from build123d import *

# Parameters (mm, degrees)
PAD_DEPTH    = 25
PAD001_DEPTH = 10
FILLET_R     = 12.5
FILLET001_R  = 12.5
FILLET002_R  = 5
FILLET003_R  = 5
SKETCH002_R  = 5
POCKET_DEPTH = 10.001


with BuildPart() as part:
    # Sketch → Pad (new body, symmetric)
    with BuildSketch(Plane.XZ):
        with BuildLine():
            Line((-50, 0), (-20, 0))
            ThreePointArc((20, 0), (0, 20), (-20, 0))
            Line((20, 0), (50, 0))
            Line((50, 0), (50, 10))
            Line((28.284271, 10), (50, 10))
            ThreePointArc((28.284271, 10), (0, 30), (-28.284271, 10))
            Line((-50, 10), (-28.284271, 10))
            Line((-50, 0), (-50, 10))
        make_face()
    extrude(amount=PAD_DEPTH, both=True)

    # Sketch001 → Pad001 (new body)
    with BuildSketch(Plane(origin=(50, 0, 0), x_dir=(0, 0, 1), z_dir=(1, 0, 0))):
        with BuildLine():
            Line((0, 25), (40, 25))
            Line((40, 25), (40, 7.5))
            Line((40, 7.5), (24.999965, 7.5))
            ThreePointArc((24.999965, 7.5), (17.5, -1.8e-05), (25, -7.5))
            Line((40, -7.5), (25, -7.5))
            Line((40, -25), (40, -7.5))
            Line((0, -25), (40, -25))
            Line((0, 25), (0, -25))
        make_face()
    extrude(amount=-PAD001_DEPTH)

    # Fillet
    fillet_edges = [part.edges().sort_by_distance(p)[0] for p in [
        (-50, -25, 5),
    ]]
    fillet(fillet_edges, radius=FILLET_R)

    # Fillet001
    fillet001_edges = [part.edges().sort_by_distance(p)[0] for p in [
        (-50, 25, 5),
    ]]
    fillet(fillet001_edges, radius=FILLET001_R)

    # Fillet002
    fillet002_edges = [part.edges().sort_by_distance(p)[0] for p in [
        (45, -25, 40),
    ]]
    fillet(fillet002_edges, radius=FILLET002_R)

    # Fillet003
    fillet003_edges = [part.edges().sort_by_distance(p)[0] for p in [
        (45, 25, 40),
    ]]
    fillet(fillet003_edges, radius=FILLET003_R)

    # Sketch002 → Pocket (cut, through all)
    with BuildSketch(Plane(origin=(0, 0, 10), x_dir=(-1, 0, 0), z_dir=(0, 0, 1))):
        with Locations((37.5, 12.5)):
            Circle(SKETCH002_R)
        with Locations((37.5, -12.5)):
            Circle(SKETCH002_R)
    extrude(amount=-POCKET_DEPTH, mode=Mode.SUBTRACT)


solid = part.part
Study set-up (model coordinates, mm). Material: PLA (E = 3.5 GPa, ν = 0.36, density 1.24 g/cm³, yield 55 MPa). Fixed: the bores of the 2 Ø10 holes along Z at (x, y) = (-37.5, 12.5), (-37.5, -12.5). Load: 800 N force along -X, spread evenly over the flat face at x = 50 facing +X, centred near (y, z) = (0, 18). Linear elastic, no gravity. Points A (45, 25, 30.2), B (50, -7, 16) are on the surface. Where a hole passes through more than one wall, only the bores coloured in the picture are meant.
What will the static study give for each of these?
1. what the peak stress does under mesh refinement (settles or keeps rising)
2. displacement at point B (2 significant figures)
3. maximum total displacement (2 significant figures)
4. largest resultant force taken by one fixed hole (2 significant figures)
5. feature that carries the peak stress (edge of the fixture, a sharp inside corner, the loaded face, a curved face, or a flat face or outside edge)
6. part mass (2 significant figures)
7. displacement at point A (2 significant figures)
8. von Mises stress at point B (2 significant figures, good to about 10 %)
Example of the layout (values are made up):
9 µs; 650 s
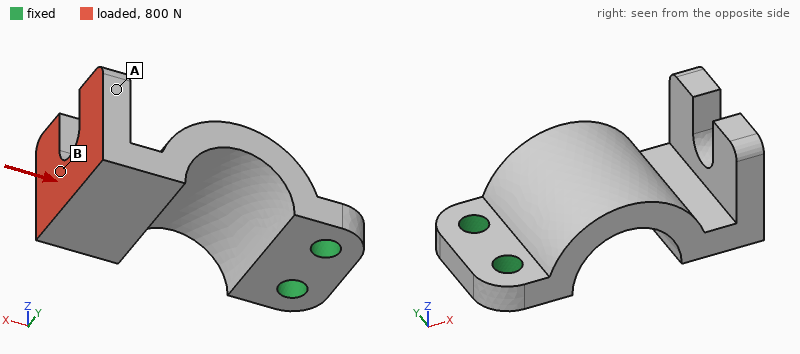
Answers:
keeps rising; 0.78 mm; 1.2 mm; 410 N; edge of the fixture; 86 g; 0.92 mm; 6.9 MPa
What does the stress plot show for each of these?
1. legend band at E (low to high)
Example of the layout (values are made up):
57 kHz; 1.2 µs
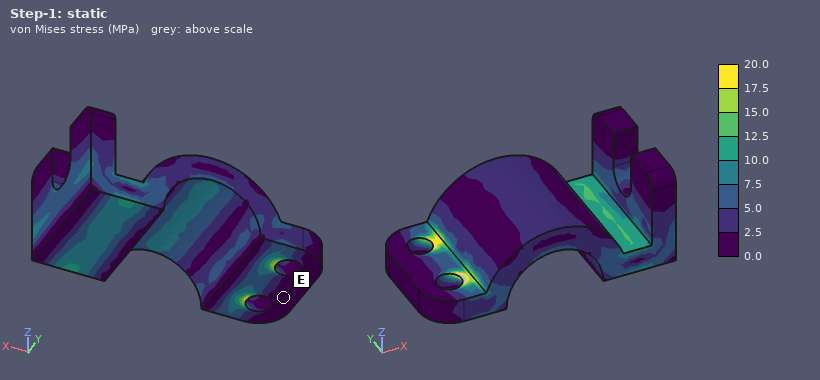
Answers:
0.0 to 2.5 MPa
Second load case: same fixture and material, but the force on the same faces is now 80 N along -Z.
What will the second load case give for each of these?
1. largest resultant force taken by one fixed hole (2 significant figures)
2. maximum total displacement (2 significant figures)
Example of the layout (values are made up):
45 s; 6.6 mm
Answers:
41 N; 1.4 mm
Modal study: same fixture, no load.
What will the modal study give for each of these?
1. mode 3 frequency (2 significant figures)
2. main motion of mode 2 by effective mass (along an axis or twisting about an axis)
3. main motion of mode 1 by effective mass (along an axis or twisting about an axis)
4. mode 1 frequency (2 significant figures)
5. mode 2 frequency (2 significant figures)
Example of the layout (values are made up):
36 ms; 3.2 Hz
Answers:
870 Hz; along Y; along Z; 240 Hz; 500 Hz
